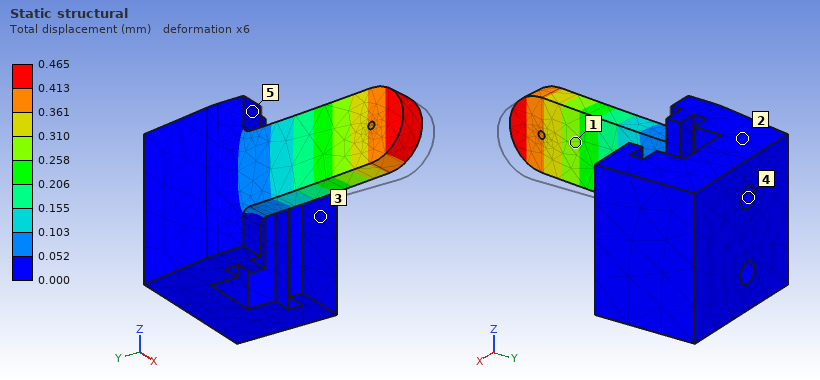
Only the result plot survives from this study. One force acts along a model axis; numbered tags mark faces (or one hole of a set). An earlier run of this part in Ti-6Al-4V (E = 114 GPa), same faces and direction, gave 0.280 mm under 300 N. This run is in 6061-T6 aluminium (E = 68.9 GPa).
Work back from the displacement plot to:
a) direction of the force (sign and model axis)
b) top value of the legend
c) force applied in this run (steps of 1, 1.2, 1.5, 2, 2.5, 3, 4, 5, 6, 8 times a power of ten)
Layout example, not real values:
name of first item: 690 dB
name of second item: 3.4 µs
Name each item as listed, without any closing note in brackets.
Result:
direction of the force: -X
top value of the legend: 0.465 mm
force applied in this run: 300 N
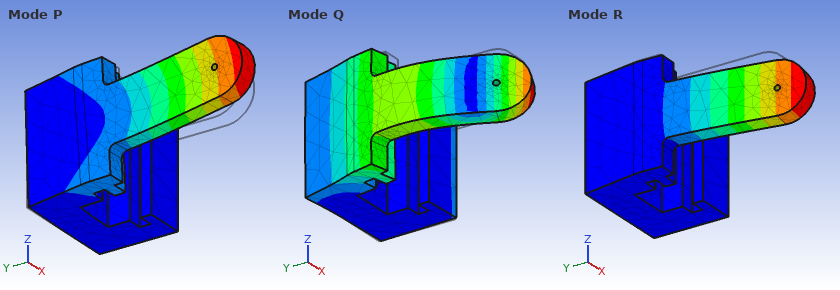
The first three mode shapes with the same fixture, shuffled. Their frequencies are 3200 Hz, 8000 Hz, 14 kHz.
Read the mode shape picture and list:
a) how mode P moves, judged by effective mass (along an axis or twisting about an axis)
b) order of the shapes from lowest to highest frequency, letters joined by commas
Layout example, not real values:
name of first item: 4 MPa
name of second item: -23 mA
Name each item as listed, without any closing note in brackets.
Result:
how mode P moves, judged by effective mass: along Z
order of the shapes from lowest to highest frequency, letters joined by commas: R, P, Q
